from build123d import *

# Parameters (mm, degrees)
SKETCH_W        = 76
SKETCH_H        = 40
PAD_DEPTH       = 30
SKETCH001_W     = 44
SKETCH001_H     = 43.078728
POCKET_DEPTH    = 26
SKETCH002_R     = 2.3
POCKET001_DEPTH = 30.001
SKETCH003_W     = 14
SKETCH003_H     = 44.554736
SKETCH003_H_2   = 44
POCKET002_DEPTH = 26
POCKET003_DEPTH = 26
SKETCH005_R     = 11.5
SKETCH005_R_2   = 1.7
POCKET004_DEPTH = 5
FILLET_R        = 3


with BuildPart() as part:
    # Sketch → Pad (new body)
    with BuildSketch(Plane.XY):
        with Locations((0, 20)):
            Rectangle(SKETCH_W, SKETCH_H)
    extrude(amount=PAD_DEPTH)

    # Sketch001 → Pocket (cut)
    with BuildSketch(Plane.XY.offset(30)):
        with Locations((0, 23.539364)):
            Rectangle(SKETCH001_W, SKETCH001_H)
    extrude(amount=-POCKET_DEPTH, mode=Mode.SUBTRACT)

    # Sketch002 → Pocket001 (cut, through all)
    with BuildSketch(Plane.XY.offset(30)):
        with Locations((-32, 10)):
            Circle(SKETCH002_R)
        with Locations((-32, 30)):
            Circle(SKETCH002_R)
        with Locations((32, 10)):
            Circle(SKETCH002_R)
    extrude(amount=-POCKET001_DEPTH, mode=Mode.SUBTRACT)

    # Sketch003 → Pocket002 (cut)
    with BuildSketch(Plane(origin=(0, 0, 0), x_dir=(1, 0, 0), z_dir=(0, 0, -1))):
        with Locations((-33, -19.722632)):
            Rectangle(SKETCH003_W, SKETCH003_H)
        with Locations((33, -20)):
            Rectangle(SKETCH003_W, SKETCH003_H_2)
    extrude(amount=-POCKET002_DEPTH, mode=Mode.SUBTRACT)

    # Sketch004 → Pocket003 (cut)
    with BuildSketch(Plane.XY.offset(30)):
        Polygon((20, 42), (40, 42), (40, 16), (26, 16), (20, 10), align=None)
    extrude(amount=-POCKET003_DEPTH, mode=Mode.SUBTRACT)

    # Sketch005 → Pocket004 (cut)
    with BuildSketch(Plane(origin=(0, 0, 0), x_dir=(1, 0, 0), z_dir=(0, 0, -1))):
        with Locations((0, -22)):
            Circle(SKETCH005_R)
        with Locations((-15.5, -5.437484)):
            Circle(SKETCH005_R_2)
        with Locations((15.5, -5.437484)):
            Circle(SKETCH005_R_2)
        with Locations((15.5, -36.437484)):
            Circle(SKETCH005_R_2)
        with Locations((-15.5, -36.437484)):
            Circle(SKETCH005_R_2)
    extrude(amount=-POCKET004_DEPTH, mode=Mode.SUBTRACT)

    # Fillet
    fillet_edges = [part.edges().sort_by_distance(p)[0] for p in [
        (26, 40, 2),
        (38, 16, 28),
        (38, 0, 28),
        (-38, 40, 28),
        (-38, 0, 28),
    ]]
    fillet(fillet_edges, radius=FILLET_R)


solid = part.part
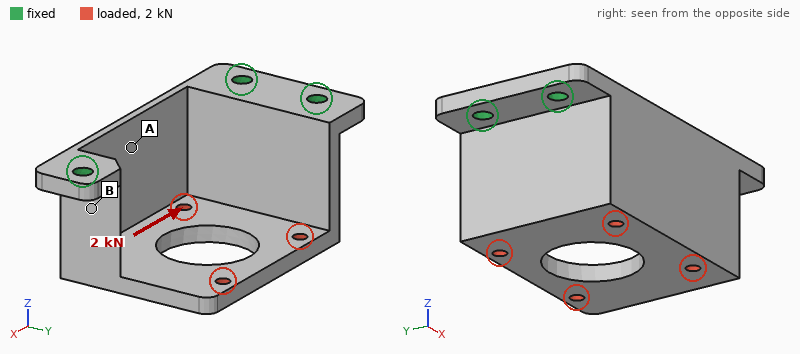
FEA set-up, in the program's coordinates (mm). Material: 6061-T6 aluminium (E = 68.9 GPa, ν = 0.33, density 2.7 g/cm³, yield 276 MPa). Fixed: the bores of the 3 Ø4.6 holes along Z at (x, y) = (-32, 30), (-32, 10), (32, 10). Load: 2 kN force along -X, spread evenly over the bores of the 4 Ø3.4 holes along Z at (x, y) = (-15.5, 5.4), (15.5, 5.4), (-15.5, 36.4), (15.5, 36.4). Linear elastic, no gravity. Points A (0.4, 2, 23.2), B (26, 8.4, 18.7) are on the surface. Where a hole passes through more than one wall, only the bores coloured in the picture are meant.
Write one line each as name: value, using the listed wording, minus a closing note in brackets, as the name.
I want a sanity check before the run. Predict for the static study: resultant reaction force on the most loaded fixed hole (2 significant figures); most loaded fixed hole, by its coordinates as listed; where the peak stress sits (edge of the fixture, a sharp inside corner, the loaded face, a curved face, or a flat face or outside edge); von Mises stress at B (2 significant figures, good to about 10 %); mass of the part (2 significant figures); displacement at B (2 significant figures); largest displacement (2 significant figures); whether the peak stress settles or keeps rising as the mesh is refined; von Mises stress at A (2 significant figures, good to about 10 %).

resultant reaction force on the most loaded fixed hole: 1.5 kN
most loaded fixed hole, by its coordinates as listed: (-32, 10)
where the peak stress sits: edge of the fixture
von Mises stress at B: 79 MPa
mass of the part: 46 g
displacement at B: 0.086 mm
largest displacement: 0.36 mm
whether the peak stress settles or keeps rising as the mesh is refined: keeps rising
von Mises stress at A: 25 MPa
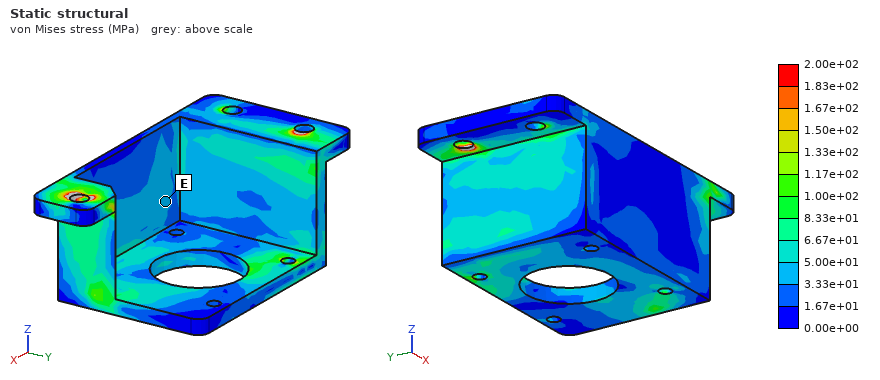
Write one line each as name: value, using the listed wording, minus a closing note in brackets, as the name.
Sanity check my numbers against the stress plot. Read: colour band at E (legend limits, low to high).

colour band at E: 3.33e+01 to 5.00e+01 MPa
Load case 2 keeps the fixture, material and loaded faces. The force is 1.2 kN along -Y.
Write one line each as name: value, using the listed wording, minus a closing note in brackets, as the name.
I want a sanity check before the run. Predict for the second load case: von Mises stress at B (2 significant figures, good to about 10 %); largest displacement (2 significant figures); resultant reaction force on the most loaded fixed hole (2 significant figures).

von Mises stress at B: 36 MPa
largest displacement: 0.21 mm
resultant reaction force on the most loaded fixed hole: 1.2 kN
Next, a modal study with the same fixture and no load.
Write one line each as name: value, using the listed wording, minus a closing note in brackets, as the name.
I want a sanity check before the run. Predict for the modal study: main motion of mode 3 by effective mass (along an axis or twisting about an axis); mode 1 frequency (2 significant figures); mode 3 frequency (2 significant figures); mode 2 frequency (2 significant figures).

main motion of mode 3 by effective mass: along Y
mode 1 frequency: 2700 Hz
mode 3 frequency: 4900 Hz
mode 2 frequency: 3600 Hz
